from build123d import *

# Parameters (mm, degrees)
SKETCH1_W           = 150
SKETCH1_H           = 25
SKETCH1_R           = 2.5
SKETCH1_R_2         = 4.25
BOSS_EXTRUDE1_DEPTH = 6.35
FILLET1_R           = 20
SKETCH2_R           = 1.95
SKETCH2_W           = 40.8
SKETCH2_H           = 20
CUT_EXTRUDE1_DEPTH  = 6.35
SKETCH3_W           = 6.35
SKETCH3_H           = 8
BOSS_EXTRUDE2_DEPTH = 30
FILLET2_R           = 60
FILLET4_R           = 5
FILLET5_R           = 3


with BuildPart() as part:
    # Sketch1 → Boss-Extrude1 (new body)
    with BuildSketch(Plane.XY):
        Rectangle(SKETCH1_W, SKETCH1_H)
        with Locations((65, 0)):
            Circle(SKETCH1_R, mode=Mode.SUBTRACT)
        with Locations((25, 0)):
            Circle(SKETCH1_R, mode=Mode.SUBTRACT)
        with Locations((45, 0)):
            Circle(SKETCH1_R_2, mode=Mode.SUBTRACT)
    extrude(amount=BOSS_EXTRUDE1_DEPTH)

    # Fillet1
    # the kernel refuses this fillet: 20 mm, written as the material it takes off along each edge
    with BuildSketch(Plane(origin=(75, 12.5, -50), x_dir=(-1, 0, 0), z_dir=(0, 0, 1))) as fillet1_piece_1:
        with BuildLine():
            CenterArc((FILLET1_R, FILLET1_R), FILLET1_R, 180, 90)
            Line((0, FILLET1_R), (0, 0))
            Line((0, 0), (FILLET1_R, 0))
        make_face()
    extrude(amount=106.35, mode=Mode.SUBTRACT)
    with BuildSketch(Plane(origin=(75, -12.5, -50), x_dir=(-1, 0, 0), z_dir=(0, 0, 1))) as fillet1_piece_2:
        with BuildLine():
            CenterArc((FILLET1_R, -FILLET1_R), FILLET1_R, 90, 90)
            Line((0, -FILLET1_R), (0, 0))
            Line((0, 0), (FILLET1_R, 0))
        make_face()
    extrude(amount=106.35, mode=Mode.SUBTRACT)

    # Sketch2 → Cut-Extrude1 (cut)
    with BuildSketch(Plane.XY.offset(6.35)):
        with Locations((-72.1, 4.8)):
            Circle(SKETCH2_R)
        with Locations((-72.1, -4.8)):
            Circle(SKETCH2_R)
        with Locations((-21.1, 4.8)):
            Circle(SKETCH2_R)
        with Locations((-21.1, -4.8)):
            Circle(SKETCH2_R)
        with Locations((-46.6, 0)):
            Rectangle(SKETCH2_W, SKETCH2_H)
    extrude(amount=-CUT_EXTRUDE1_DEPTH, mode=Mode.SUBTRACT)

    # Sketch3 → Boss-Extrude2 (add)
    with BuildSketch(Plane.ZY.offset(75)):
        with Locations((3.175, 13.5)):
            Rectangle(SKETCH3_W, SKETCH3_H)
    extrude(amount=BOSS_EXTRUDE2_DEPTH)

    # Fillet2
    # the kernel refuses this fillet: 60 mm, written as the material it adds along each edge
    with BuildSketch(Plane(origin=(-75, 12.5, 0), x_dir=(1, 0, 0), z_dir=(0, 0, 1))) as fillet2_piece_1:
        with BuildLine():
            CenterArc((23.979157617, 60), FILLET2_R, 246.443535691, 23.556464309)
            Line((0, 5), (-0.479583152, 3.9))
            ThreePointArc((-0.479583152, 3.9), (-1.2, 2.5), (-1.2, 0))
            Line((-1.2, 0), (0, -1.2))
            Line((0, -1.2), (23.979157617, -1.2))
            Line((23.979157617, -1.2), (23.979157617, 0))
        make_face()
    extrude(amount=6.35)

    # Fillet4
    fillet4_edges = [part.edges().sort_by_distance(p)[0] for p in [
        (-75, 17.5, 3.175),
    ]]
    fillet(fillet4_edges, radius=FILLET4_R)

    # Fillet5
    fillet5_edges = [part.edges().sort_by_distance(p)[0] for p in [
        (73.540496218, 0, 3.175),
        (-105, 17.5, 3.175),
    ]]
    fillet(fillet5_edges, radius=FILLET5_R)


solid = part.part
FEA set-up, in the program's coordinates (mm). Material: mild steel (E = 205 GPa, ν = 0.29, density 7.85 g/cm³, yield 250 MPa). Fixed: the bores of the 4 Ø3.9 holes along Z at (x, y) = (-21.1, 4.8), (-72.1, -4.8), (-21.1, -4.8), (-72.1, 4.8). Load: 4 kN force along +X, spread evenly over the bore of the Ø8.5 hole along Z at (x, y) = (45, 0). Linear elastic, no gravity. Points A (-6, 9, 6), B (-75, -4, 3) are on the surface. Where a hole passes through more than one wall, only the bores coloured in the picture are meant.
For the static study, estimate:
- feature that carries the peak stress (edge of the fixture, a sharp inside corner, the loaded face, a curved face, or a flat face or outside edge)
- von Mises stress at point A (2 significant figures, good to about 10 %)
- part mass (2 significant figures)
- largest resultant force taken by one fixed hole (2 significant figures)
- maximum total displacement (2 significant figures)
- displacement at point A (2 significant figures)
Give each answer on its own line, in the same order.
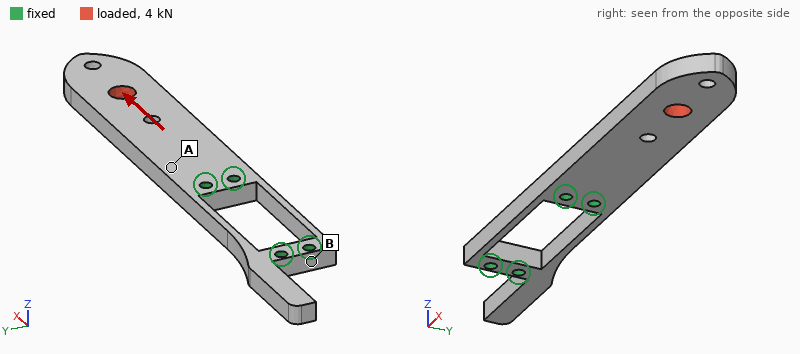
a curved face
24 MPa
140 g
2.0 kN
9.9 µm
2.1 µm
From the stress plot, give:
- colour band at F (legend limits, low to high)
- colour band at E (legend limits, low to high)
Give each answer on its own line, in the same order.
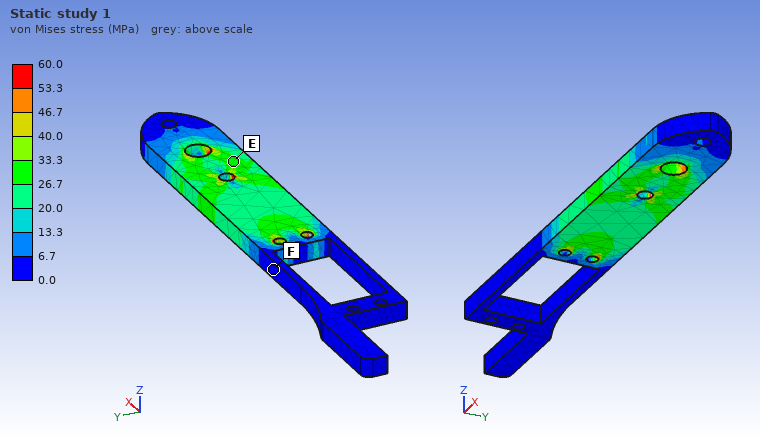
0.0 to 6.7 MPa
26.7 to 33.3 MPa
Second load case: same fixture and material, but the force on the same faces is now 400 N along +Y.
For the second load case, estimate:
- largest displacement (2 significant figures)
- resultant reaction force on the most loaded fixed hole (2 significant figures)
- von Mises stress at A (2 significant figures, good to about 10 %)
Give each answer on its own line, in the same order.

48 µm
1.9 kN
22 MPa
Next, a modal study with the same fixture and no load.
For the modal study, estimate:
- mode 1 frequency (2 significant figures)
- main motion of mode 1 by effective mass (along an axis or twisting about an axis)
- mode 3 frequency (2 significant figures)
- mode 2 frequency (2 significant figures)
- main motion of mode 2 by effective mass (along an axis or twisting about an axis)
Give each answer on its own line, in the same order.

680 Hz
along Z
3600 Hz
2300 Hz
along Y
